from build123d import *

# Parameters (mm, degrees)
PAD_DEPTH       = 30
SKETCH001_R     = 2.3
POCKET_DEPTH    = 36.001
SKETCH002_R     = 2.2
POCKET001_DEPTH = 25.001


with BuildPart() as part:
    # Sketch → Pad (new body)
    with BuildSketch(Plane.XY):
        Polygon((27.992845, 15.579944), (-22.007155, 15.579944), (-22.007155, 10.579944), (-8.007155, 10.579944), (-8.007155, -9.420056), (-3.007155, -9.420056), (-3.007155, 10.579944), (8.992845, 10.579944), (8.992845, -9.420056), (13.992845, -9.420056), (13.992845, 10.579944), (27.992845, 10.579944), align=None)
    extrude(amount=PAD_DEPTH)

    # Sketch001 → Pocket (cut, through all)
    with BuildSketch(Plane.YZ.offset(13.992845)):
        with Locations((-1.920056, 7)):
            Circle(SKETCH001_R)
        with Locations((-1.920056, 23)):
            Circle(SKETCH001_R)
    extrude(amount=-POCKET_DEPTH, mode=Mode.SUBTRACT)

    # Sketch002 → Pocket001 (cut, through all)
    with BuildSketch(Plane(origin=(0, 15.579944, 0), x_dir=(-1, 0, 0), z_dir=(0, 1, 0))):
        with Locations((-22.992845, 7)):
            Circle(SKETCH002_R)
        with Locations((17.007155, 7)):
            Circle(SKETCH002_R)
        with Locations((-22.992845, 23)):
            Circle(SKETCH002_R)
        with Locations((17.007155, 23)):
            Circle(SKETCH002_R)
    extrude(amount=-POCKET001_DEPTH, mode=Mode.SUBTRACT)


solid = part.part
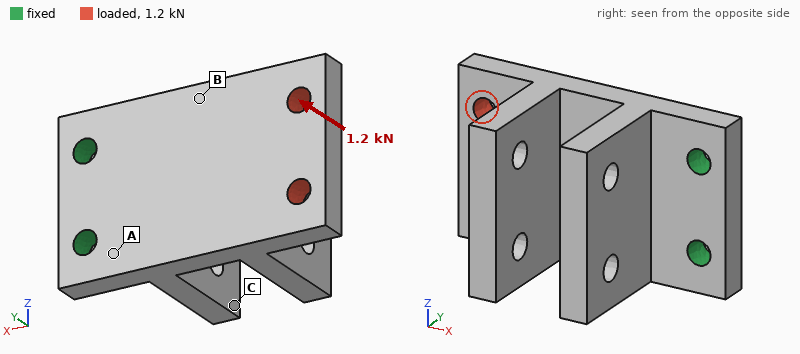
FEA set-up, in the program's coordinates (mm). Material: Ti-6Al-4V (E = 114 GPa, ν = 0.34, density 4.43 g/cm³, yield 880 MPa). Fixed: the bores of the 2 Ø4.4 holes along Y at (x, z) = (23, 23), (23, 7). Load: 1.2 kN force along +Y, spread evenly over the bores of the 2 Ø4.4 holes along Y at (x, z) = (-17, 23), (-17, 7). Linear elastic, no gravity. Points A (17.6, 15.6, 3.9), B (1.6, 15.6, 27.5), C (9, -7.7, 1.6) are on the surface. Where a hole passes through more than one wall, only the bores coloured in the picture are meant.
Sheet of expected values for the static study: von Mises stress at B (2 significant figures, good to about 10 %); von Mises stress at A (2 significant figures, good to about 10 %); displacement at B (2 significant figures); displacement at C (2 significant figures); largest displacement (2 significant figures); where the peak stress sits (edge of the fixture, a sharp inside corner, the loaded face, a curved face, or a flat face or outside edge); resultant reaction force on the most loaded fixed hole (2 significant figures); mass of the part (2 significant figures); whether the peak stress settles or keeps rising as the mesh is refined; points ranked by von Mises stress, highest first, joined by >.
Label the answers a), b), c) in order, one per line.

a) 170 MPa
b) 310 MPa
c) 0.22 mm
d) 0.25 mm
e) 0.73 mm
f) edge of the fixture
g) 600 N
h) 57 g
i) keeps rising
j) A > B > C
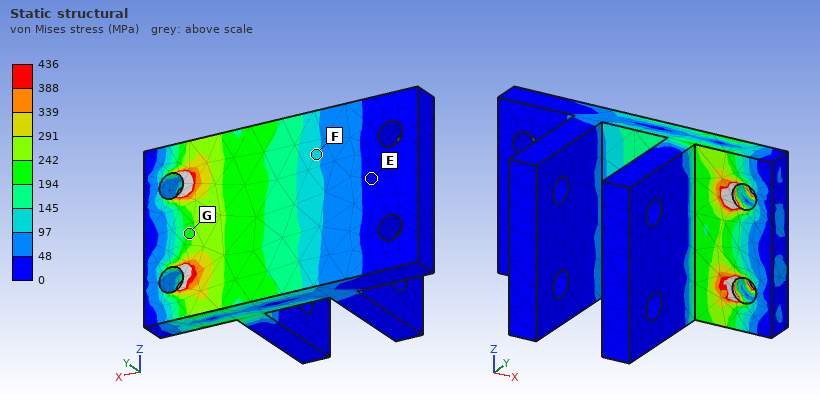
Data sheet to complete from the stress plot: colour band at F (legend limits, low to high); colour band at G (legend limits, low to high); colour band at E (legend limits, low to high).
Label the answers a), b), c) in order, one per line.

a) 97 to 145 MPa
b) 194 to 242 MPa
c) 0 to 48 MPa
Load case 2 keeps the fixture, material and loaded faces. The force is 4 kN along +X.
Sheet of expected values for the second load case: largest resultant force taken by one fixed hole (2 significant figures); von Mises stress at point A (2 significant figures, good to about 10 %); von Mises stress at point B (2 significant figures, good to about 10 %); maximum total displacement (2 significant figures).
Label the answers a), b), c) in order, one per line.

a) 2.0 kN
b) 29 MPa
c) 27 MPa
d) 14 µm
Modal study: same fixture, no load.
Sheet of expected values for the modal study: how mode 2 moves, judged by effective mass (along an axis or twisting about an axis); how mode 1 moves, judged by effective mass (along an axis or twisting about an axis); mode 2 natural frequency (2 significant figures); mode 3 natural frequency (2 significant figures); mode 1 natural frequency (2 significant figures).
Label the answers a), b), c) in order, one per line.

a) along Z
b) along Y
c) 4100 Hz
d) 5800 Hz
e) 1700 Hz
